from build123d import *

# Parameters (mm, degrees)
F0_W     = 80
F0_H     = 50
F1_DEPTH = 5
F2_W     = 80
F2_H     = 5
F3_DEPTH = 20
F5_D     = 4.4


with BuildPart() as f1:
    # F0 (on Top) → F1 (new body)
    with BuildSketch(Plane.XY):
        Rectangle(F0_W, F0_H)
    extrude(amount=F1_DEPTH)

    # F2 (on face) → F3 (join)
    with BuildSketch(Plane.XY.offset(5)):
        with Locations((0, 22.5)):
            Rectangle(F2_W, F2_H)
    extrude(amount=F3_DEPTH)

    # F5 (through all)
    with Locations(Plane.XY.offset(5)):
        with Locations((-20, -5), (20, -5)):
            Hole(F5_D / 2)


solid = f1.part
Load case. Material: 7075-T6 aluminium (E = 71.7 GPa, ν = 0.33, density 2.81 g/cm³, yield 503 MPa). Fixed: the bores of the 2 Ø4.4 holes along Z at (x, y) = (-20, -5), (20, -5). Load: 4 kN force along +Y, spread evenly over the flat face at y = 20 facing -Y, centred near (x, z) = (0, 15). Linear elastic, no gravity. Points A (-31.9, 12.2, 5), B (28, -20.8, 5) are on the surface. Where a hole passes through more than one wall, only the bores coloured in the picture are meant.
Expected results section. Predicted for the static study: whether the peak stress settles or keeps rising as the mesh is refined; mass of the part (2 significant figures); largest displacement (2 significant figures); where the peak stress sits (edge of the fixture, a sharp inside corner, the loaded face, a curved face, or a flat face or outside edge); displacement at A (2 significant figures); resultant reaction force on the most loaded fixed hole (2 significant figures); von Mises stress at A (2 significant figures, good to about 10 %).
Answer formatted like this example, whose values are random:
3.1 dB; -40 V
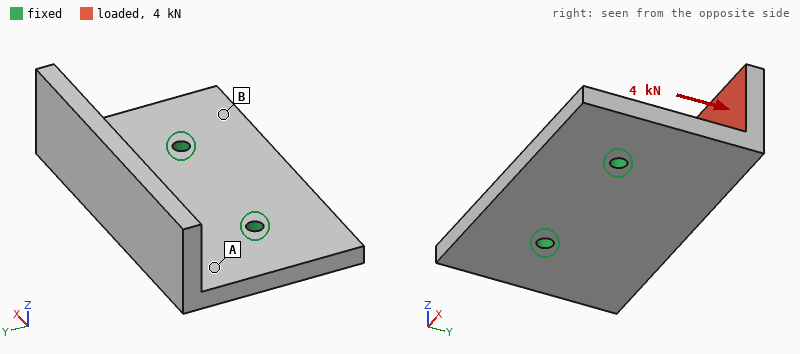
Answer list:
keeps rising; 78 g; 0.75 mm; edge of the fixture; 0.16 mm; 2.0 kN; 140 MPa
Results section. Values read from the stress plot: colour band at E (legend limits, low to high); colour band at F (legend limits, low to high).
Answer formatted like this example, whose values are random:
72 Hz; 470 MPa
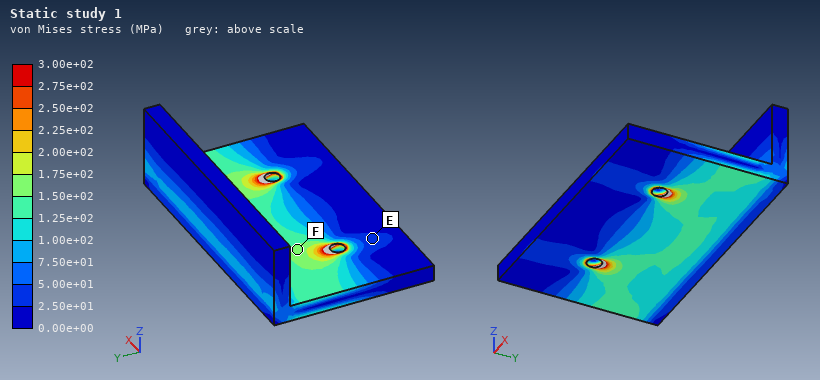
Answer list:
2.50e+01 to 5.00e+01 MPa; 1.50e+02 to 1.75e+02 MPa
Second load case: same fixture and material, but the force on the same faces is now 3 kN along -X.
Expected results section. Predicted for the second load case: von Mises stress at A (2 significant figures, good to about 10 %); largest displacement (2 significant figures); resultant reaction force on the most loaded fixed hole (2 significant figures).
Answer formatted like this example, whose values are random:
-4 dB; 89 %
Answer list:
36 MPa; 0.26 mm; 2.4 kN
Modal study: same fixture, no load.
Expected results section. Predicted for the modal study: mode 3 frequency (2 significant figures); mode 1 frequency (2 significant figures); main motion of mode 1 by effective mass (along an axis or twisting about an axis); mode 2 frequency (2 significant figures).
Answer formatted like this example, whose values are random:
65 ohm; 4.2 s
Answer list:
6000 Hz; 1900 Hz; along Z; 2900 Hz
